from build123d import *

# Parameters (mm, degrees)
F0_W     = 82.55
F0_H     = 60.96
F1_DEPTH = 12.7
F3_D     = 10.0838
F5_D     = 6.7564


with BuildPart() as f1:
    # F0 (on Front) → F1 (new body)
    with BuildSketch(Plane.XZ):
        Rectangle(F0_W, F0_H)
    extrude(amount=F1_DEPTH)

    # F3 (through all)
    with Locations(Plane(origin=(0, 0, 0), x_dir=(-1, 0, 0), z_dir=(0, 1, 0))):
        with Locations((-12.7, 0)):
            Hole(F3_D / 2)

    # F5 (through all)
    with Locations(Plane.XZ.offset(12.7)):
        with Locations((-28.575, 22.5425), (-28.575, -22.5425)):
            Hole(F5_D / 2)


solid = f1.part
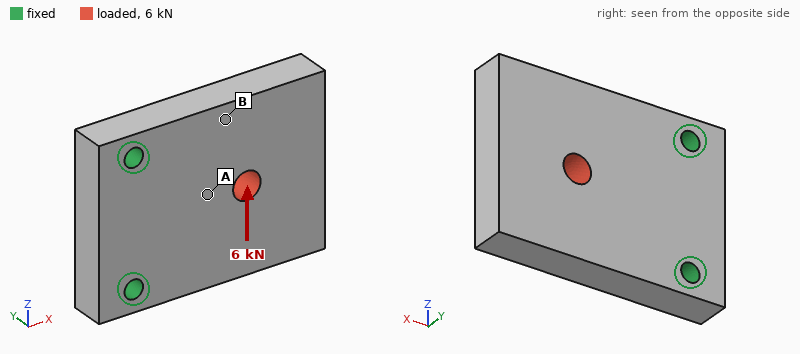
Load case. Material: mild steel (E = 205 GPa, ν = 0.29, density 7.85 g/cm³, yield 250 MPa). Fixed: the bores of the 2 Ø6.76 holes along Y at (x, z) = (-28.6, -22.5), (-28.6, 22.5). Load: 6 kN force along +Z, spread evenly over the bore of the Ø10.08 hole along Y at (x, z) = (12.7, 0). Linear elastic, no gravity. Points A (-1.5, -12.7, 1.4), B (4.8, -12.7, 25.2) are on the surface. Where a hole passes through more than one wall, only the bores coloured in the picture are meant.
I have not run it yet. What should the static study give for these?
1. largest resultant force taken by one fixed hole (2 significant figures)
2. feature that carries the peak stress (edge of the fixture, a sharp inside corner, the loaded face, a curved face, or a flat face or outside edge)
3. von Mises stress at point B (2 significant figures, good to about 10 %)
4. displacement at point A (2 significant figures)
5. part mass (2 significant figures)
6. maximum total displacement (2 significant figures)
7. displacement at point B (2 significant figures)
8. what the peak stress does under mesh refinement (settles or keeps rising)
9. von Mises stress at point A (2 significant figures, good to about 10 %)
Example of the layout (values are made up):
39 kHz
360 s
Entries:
5.9 kN
edge of the fixture
8.2 MPa
4.5 µm
490 g
12 µm
6.4 µm
keeps rising
22 MPa
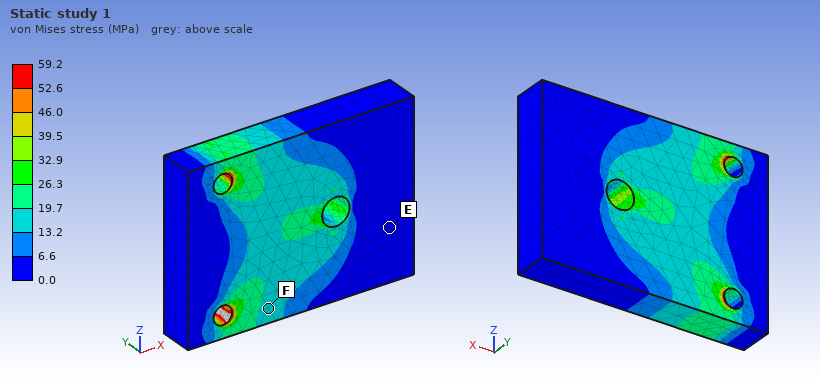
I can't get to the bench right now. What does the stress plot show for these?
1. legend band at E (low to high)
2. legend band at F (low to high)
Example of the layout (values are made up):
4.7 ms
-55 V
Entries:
0.0 to 6.6 MPa
13.2 to 19.7 MPa
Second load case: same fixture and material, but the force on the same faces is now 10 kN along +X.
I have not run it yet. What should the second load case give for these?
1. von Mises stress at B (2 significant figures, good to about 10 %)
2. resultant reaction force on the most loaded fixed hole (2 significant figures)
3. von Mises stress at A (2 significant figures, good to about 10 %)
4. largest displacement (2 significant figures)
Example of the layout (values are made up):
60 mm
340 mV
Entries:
8.0 MPa
5.1 kN
19 MPa
5.0 µm
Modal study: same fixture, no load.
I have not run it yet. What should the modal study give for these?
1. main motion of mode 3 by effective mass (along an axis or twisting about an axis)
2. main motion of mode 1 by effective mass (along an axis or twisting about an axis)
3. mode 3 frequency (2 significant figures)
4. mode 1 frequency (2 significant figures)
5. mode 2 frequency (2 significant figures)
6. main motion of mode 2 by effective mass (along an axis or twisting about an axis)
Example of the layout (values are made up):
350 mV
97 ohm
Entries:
along Z
along Y
7000 Hz
2000 Hz
5200 Hz
twisting about X
